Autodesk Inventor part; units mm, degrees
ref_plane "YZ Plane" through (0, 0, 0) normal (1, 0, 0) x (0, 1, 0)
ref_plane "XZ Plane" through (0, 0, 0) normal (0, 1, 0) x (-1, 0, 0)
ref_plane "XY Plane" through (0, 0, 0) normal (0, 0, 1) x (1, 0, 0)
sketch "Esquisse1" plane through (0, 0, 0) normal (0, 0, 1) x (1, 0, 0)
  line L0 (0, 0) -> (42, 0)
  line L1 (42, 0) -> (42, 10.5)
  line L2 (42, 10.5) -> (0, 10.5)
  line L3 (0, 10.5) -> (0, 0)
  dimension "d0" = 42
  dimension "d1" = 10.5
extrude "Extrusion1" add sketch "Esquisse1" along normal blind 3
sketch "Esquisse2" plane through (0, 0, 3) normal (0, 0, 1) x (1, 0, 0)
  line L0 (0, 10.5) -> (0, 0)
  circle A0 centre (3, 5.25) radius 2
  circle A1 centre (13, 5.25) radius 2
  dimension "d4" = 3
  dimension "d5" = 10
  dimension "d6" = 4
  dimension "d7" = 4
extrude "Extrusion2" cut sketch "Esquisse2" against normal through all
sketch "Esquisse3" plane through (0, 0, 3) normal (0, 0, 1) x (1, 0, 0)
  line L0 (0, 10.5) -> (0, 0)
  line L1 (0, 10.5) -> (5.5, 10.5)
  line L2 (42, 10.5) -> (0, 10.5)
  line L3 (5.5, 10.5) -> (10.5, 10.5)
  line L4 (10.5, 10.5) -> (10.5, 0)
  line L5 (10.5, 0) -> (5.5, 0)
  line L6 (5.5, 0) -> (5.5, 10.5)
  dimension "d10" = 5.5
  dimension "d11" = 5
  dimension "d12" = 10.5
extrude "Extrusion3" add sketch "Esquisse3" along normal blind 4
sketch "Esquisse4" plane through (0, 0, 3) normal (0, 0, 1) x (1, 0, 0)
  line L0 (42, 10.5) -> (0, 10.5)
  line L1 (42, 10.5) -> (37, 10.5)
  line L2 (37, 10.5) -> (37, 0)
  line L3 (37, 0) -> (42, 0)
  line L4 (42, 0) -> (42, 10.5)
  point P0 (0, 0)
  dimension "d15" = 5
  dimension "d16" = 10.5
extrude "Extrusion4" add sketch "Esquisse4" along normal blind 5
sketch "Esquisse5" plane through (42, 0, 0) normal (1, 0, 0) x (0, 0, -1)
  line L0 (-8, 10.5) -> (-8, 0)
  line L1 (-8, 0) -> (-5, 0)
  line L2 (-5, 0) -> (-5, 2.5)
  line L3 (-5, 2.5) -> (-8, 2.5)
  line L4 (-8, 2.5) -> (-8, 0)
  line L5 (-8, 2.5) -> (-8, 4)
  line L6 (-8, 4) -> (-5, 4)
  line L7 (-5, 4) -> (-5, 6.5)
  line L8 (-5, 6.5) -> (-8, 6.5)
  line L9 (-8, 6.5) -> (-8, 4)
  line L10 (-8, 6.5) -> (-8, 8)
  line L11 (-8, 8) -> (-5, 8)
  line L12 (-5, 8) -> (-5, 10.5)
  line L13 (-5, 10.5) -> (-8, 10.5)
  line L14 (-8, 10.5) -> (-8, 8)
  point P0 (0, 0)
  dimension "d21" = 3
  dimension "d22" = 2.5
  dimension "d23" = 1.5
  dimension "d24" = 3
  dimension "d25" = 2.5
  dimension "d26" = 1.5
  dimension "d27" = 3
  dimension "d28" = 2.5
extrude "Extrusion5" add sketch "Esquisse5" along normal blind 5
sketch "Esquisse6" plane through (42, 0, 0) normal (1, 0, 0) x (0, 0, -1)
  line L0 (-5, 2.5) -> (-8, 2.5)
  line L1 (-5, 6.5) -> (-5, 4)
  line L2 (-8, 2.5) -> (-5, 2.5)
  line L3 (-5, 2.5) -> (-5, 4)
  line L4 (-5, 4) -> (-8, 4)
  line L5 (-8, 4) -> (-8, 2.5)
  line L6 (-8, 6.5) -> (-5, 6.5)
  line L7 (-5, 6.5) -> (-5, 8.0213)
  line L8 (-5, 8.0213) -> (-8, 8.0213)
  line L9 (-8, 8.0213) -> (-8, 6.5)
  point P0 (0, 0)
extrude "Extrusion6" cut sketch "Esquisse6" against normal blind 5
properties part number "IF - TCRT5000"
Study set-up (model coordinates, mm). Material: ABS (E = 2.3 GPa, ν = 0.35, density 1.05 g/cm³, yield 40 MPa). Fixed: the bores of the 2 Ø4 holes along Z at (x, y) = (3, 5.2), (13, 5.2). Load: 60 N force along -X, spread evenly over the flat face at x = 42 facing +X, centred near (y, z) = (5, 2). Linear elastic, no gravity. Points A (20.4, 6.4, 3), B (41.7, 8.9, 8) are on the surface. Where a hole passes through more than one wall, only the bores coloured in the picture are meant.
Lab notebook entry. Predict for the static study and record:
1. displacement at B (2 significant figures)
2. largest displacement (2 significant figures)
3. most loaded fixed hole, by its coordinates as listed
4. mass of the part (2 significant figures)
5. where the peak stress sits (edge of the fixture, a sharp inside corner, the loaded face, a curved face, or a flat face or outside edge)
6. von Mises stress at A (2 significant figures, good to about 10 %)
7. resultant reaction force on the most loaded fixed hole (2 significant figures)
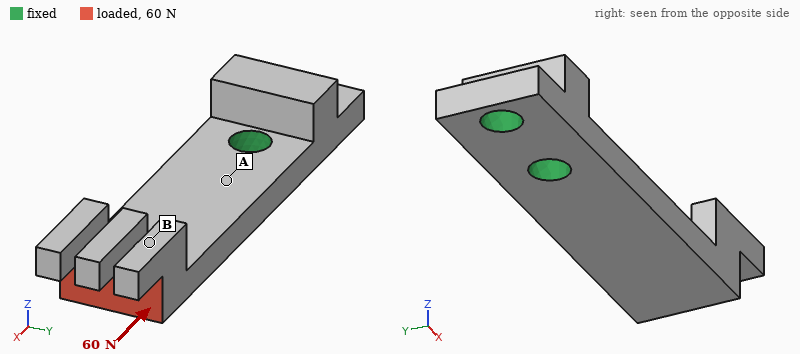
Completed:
0.45 mm
0.57 mm
(13, 5.2)
1.9 g
a flat face or outside edge
5.8 MPa
54 N
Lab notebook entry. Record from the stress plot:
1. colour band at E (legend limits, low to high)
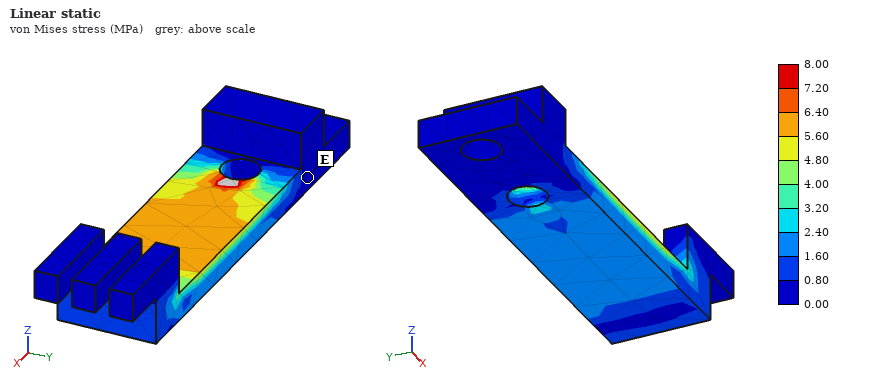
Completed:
0.00 to 0.80 MPa
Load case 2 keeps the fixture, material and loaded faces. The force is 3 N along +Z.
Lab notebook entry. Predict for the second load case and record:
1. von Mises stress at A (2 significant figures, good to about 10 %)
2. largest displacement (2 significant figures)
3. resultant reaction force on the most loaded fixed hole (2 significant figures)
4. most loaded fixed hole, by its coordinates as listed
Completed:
3.9 MPa
0.51 mm
3.6 N
(13, 5.2)
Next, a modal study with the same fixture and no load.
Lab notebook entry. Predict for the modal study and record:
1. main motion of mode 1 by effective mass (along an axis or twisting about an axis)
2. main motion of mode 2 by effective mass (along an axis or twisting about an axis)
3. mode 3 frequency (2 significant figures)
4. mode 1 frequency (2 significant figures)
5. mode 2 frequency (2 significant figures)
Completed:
along Z
along Y
2800 Hz
590 Hz
1500 Hz
